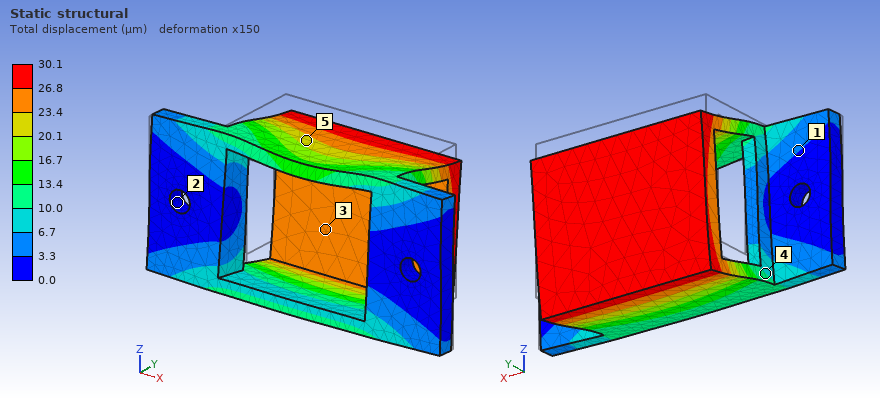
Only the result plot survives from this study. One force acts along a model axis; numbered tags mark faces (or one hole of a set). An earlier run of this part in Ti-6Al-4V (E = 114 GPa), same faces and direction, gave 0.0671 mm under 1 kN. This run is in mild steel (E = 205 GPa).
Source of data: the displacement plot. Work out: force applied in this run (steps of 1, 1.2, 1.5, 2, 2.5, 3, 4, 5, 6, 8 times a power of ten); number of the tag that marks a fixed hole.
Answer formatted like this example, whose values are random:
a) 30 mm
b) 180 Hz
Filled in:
a) 800 N
b) 2
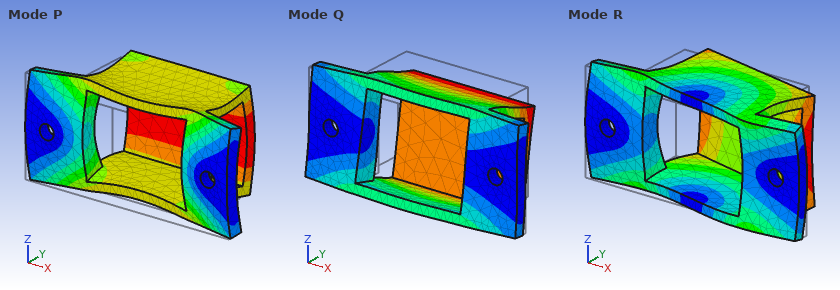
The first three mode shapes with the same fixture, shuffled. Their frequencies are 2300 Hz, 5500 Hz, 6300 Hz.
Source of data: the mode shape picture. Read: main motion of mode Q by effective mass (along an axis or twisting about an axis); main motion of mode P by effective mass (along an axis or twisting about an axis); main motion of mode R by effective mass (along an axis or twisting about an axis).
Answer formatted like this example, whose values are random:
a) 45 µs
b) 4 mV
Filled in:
a) along Z
b) along Y
c) along X
